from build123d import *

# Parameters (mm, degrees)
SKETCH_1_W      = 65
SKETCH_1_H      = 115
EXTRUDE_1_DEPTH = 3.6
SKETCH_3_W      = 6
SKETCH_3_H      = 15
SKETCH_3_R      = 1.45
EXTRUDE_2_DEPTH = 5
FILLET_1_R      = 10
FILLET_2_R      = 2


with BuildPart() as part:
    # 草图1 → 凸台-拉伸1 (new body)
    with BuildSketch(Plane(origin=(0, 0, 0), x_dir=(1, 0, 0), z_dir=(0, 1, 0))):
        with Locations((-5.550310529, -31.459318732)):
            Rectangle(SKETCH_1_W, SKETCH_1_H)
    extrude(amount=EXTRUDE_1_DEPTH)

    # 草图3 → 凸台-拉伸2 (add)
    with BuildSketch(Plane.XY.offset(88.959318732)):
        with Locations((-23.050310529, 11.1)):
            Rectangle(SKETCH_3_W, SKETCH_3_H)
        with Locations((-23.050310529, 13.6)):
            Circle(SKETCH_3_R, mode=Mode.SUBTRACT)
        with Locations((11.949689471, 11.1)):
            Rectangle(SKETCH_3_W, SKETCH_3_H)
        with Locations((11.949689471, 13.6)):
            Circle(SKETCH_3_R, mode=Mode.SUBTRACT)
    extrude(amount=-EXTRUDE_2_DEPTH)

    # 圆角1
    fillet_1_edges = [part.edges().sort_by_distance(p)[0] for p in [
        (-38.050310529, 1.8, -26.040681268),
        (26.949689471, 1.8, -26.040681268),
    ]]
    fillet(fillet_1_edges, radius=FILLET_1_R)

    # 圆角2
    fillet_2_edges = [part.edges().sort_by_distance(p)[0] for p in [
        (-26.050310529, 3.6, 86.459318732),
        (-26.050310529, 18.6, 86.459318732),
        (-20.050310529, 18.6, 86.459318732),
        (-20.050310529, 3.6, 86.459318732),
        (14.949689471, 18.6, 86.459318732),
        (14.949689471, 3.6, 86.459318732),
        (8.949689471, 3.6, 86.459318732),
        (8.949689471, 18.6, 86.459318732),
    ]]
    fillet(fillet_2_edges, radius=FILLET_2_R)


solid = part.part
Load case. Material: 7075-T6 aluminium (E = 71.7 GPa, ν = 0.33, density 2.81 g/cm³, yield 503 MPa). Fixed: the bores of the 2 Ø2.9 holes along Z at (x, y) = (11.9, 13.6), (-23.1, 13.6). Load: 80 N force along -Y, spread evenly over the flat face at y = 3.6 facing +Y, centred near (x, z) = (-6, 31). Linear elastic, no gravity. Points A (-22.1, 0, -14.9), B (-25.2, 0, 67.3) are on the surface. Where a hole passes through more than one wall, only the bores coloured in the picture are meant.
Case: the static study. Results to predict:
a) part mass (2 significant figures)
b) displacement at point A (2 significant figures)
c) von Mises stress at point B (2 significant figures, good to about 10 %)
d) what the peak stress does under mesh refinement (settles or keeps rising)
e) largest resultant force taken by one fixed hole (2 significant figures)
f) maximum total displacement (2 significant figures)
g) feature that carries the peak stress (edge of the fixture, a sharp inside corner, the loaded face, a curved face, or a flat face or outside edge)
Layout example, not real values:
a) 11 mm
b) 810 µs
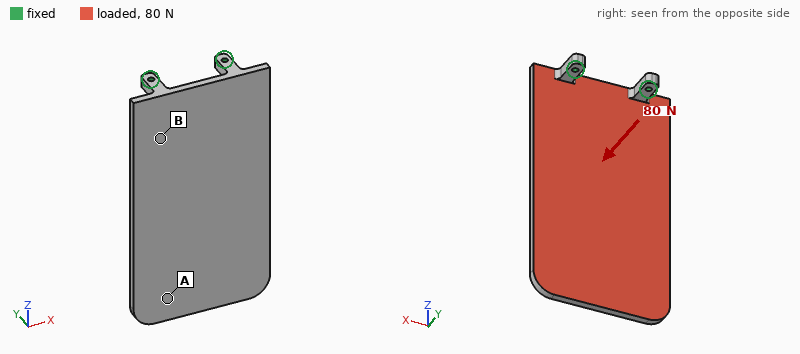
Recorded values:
a) 78 g
b) 1.2 mm
c) 20 MPa
d) keeps rising
e) 47 N
f) 1.4 mm
g) edge of the fixture
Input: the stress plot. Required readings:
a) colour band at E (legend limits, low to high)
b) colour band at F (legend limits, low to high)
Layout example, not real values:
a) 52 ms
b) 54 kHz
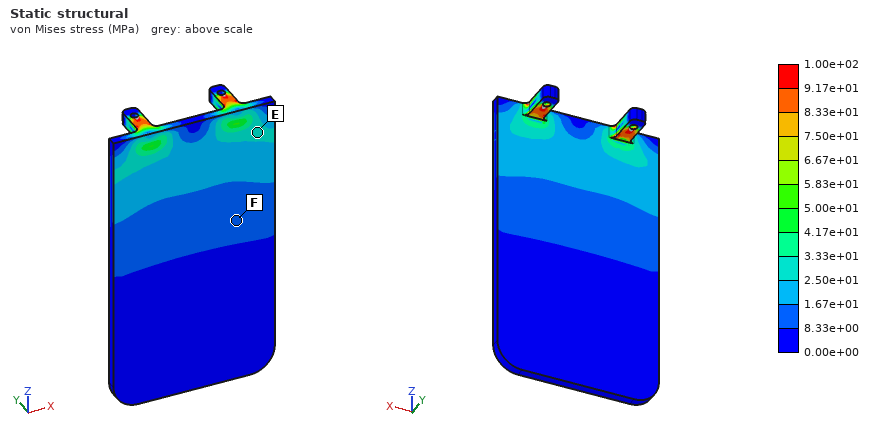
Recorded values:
a) 2.50e+01 to 3.33e+01 MPa
b) 8.33e+00 to 1.67e+01 MPa
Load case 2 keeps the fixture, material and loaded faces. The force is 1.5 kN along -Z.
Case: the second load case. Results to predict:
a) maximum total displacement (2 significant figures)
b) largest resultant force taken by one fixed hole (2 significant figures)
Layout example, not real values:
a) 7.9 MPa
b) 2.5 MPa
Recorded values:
a) 0.22 mm
b) 750 N
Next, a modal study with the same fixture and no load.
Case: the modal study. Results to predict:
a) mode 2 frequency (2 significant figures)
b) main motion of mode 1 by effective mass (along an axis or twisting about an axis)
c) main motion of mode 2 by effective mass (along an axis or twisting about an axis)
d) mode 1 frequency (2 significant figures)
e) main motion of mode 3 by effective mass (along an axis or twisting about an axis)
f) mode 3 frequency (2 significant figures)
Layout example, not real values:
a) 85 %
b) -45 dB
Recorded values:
a) 730 Hz
b) along Y
c) along X
d) 170 Hz
e) along X
f) 930 Hz
